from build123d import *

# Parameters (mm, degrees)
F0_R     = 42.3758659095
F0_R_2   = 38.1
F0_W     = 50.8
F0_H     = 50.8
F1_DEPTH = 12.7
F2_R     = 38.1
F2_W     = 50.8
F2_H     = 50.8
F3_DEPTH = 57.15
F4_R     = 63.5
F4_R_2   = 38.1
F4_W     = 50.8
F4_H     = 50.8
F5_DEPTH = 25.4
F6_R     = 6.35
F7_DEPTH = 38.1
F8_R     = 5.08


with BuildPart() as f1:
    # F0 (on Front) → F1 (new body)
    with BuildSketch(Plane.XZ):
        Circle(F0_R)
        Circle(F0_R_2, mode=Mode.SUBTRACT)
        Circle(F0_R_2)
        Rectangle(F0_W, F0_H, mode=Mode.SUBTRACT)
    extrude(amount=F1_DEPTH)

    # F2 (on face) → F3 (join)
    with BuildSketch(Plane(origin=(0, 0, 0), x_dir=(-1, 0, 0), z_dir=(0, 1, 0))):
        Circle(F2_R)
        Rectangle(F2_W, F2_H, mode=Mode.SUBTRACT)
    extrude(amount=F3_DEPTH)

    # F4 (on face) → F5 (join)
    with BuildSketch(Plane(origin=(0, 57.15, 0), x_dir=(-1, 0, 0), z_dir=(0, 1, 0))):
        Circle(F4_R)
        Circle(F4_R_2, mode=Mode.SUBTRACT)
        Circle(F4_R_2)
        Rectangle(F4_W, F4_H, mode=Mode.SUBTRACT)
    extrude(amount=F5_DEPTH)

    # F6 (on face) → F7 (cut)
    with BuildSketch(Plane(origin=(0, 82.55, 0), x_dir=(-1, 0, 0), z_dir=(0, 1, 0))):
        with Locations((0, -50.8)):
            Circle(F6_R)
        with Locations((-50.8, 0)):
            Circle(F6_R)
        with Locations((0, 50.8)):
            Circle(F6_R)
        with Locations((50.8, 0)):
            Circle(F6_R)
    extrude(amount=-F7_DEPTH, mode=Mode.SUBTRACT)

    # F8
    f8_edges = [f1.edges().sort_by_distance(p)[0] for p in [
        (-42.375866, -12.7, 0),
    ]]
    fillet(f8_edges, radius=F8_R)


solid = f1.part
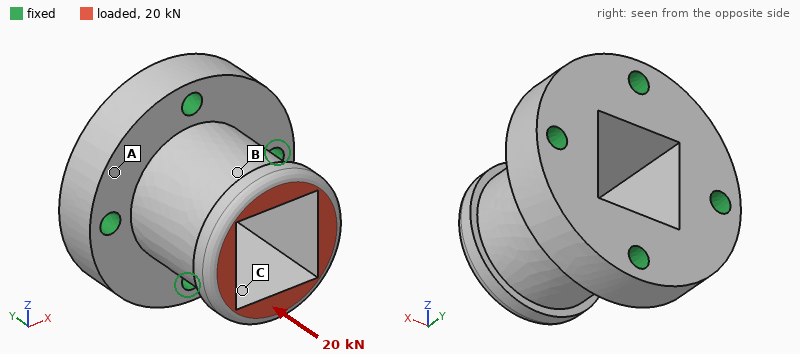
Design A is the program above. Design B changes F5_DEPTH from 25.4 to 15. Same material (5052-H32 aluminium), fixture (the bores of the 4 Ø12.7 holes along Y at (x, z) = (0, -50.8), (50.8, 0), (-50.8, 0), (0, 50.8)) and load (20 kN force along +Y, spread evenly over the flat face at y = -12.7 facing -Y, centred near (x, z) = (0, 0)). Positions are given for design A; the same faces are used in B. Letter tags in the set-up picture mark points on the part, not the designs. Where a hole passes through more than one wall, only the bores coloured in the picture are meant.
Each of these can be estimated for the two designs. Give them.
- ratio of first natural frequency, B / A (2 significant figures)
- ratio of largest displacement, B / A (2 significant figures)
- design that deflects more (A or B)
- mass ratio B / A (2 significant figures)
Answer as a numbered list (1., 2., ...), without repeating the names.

1. 0.90
2. 1.3
3. B
4. 0.75
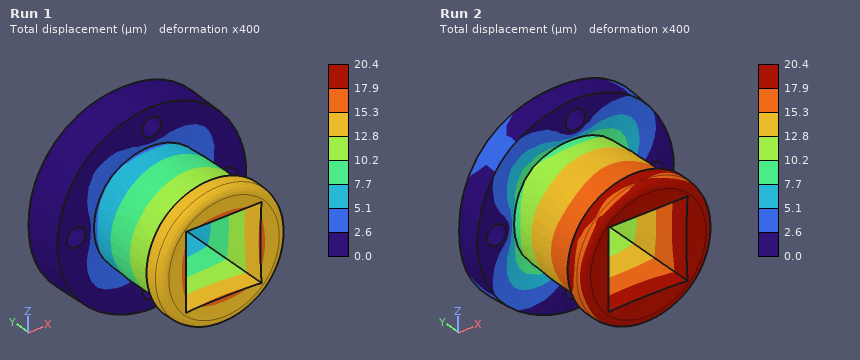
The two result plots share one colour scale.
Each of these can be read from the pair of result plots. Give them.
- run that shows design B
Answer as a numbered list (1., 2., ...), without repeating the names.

1. Run 2
